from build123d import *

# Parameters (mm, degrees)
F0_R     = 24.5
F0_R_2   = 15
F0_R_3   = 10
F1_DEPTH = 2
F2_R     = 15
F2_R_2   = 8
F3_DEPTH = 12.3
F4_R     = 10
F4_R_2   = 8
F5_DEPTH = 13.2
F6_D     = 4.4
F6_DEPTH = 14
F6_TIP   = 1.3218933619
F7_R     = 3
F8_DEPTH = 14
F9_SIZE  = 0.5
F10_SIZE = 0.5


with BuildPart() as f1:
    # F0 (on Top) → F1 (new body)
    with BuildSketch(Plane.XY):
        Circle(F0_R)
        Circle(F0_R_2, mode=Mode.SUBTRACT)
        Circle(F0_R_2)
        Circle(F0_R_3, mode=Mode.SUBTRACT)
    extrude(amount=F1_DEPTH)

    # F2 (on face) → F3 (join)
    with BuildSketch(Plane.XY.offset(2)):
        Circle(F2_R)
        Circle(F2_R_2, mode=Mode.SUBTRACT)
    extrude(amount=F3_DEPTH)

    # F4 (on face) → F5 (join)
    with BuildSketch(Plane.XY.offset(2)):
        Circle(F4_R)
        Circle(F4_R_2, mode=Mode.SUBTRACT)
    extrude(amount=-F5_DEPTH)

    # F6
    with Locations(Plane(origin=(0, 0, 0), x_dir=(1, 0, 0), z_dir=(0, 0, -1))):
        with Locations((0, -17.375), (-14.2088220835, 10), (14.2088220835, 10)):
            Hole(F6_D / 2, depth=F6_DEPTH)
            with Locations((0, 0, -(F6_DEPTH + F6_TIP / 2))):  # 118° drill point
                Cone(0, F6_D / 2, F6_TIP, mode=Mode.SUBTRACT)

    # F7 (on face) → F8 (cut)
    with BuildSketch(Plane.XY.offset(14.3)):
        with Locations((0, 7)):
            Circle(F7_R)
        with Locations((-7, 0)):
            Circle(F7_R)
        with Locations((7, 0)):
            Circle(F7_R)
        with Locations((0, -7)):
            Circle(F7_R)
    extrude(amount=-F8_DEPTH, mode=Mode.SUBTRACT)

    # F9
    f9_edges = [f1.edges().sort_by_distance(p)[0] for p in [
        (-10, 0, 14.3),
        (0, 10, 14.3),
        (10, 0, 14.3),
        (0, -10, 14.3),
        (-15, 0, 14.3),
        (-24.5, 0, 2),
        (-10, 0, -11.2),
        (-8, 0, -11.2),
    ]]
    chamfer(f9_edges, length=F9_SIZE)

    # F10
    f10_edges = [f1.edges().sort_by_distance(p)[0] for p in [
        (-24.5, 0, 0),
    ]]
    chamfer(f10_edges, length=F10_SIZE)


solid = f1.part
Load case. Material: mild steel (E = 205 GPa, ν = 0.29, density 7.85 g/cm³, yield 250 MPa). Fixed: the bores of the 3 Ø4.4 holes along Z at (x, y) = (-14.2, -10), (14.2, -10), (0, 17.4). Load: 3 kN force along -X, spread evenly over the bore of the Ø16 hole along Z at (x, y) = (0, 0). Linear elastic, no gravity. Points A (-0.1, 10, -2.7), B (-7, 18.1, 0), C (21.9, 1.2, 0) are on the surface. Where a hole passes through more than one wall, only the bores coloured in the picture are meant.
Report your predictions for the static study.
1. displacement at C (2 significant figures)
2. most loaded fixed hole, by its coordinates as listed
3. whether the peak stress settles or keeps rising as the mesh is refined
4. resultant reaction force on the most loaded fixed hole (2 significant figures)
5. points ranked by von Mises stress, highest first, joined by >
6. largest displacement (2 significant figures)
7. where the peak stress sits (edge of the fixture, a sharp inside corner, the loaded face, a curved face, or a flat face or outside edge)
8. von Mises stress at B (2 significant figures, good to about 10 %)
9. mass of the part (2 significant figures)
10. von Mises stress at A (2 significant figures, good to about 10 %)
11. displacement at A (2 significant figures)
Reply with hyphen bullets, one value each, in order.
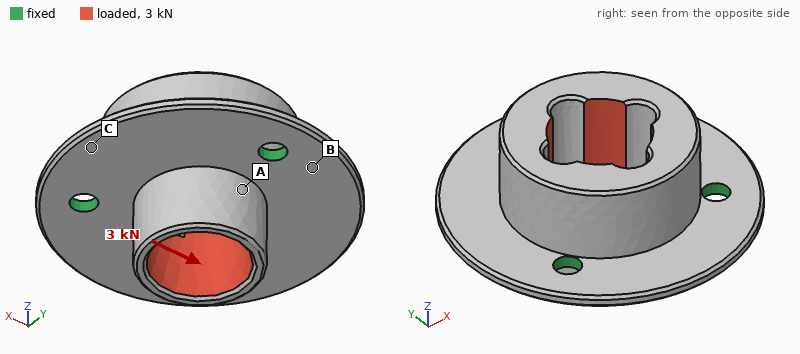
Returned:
- 1.8 µm
- (0, 17.4)
- keeps rising
- 1.2 kN
- A > B > C
- 6.9 µm
- edge of the fixture
- 19 MPa
- 80 g
- 28 MPa
- 3.4 µm
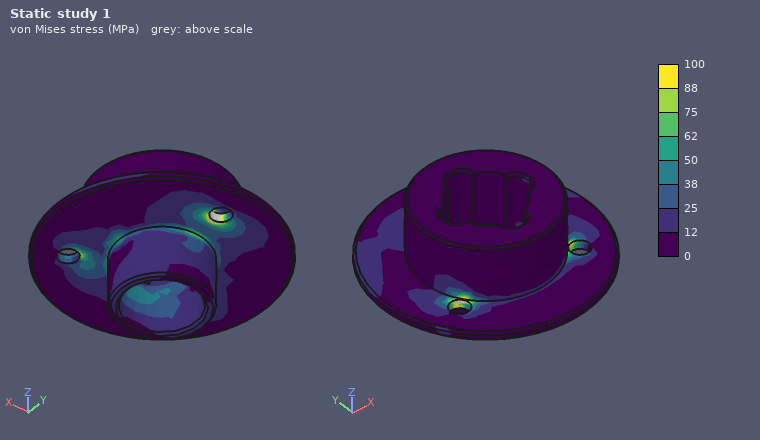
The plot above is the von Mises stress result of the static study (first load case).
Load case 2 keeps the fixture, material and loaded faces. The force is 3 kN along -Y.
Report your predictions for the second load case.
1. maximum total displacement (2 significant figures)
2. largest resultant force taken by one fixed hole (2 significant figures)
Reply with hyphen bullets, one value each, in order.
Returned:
- 6.8 µm
- 1.1 kN
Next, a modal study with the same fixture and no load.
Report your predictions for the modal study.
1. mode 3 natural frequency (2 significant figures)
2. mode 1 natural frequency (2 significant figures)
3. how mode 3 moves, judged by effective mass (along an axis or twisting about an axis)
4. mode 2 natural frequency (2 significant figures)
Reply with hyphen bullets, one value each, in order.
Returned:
- 15 kHz
- 12 kHz
- along Z
- 13 kHz
